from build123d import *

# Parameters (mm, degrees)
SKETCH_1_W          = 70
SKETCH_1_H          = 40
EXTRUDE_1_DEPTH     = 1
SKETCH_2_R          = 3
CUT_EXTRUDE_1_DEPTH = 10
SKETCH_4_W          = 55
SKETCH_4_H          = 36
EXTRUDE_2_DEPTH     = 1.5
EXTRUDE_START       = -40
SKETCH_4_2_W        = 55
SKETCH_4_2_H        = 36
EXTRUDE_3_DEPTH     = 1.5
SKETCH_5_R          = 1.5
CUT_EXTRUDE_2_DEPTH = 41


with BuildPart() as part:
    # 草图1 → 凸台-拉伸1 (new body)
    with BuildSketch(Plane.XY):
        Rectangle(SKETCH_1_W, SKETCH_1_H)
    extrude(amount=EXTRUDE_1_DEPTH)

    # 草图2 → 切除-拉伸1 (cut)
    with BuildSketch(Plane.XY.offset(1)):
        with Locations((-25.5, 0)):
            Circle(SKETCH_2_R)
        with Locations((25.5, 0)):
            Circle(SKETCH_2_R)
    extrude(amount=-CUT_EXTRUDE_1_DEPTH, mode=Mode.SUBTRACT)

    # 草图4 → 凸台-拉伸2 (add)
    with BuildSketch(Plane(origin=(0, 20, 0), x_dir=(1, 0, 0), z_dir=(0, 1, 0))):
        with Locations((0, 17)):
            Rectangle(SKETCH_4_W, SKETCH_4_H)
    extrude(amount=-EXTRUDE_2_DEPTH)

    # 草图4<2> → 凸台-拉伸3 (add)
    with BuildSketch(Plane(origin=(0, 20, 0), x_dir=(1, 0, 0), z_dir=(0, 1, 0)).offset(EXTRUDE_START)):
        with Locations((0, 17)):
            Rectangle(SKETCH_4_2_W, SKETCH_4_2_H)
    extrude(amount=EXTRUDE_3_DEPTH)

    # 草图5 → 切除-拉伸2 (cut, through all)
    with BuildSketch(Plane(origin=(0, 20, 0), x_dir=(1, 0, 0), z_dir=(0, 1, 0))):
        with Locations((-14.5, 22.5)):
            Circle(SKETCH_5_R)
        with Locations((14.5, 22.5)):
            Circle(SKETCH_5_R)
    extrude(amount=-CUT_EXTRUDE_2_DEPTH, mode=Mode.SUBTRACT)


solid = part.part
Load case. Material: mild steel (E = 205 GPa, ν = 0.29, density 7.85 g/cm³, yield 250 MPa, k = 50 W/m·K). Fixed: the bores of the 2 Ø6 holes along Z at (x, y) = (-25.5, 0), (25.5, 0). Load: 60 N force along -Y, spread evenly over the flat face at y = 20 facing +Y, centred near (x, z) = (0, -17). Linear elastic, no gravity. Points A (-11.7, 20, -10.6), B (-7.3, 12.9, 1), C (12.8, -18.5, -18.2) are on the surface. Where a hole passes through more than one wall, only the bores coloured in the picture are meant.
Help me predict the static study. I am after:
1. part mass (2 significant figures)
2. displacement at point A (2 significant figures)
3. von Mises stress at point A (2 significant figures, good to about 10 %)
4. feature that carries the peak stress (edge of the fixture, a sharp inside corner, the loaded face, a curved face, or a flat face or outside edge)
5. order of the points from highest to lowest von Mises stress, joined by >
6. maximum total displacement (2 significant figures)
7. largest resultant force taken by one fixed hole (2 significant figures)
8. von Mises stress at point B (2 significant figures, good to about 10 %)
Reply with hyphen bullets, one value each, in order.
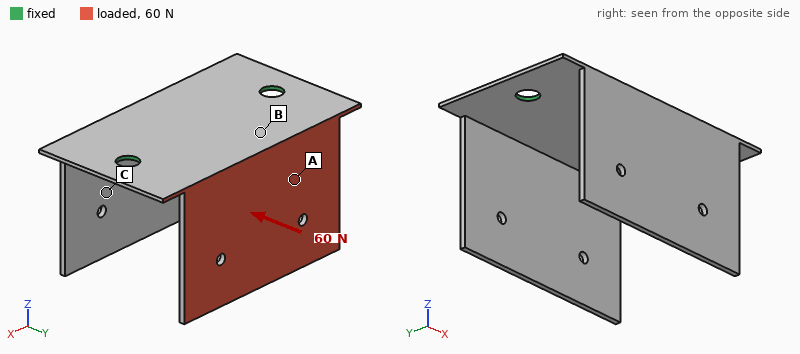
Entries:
- 67 g
- 0.24 mm
- 21 MPa
- a flat face or outside edge
- B > A > C
- 0.66 mm
- 30 N
- 83 MPa
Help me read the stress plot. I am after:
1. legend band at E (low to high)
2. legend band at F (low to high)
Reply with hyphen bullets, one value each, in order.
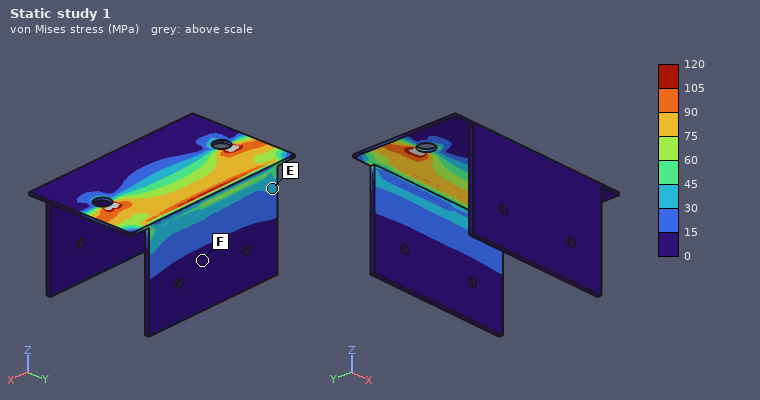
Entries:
- 30 to 45 MPa
- 0 to 15 MPa
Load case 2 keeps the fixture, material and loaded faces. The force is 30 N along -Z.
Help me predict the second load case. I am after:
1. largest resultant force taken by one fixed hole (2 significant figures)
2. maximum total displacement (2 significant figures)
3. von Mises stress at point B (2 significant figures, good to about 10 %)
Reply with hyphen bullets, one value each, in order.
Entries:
- 15 N
- 0.18 mm
- 16 MPa
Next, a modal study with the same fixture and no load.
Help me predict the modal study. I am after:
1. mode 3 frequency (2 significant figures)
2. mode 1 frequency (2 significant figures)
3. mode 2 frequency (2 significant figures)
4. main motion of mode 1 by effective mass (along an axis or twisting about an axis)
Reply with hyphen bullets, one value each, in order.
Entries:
- 930 Hz
- 350 Hz
- 370 Hz
- along Y
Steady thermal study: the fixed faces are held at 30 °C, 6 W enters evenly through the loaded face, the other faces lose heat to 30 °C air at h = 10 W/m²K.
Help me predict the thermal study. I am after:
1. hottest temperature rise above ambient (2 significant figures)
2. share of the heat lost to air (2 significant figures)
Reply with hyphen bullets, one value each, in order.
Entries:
- 54 K
- 31 %
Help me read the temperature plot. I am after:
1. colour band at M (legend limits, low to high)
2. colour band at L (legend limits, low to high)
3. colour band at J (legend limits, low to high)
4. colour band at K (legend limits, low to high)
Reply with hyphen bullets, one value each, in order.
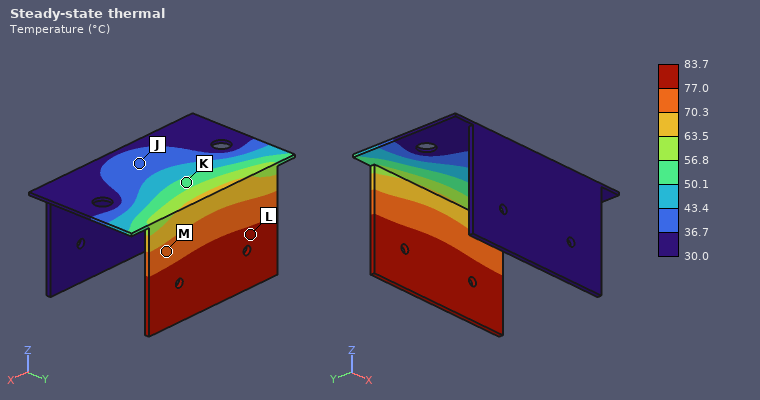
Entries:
- 70.3 to 77.0 °C
- 77.0 to 83.7 °C
- 36.7 to 43.4 °C
- 50.1 to 56.8 °C
